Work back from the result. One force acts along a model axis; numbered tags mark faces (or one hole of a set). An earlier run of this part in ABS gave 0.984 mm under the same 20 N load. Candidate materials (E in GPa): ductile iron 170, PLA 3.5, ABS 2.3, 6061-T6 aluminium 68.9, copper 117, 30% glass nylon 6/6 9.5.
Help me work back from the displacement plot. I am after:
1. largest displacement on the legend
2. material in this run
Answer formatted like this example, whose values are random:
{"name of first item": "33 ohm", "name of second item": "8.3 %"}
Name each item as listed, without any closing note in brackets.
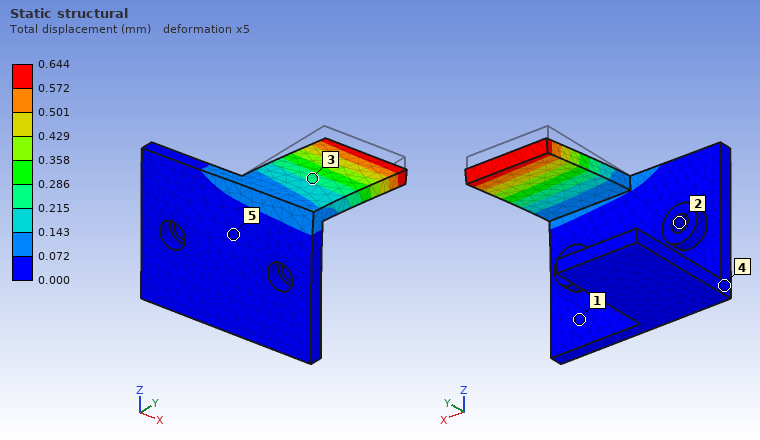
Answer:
{"largest displacement on the legend": "0.644 mm", "material in this run": "PLA"}
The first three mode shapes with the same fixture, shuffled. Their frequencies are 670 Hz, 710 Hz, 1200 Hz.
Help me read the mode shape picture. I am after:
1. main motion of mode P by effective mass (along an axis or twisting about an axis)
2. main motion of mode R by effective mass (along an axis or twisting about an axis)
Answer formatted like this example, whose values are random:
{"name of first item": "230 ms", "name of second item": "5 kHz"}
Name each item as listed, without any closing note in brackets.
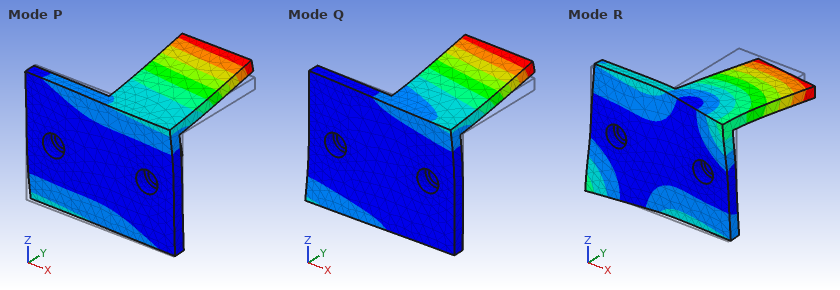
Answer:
{"main motion of mode P by effective mass": "along Z", "main motion of mode R by effective mass": "twisting about Y"}
